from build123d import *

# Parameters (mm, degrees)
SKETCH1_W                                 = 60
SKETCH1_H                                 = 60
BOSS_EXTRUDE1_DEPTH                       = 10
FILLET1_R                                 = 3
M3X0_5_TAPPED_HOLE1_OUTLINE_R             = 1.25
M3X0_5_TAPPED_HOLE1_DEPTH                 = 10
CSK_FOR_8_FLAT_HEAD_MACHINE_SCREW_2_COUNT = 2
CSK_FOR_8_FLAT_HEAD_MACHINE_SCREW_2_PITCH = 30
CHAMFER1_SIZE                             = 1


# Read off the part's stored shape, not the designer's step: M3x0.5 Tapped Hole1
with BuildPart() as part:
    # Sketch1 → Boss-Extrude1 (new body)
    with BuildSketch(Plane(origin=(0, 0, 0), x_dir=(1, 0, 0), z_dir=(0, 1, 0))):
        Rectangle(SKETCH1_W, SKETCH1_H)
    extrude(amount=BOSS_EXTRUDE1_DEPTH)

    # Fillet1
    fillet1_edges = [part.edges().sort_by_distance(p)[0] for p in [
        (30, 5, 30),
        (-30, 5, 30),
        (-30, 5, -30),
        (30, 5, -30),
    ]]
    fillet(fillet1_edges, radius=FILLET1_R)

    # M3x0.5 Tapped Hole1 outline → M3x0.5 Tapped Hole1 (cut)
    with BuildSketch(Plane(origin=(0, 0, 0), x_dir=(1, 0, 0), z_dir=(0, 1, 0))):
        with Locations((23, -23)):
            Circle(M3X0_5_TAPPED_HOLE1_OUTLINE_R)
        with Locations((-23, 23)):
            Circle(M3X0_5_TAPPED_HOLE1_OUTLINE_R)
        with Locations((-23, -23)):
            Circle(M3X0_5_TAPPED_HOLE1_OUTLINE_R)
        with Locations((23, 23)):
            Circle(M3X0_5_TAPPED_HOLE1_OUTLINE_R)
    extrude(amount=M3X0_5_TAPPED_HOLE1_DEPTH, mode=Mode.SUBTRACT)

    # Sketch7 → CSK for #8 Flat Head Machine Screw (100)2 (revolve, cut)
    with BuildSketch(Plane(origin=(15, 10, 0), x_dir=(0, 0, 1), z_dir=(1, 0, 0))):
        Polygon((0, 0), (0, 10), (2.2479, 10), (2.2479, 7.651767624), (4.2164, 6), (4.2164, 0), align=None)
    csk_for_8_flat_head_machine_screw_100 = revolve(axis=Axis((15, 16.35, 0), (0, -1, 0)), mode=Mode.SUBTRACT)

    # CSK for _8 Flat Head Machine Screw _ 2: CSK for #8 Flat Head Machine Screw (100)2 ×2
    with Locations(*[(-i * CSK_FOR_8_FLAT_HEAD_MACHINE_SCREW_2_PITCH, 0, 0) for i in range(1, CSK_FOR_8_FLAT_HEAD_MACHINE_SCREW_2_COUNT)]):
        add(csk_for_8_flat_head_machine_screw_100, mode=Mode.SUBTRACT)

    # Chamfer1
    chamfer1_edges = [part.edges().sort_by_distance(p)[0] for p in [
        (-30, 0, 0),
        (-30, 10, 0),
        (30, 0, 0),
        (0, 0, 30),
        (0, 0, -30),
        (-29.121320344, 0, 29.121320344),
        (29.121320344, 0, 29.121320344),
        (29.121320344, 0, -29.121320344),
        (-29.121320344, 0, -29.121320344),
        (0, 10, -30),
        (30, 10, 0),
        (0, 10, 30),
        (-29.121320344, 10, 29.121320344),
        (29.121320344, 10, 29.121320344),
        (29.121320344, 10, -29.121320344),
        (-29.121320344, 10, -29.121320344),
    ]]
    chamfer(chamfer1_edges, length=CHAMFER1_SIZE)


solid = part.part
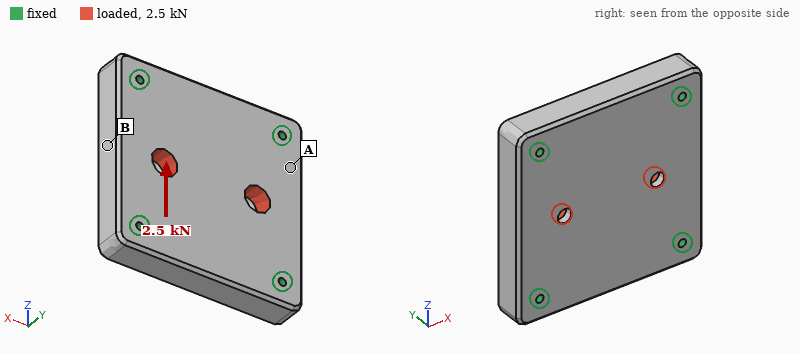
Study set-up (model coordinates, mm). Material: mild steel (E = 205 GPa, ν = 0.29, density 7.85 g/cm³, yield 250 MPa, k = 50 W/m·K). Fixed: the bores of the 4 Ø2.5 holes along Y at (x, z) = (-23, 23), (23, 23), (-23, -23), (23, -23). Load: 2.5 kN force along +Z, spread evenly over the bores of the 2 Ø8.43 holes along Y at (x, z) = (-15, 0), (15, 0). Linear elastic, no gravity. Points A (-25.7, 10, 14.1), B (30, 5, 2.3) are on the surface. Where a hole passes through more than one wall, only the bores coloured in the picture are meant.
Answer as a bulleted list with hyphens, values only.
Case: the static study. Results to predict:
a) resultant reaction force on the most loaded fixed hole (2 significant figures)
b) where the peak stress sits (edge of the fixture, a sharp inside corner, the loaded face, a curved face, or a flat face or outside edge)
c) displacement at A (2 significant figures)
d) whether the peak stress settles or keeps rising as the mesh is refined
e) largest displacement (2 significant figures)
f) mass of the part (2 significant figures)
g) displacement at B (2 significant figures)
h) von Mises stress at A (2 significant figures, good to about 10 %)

- 650 N
- edge of the fixture
- 0.19 µm
- keeps rising
- 0.75 µm
- 270 g
- 0.25 µm
- 3.8 MPa
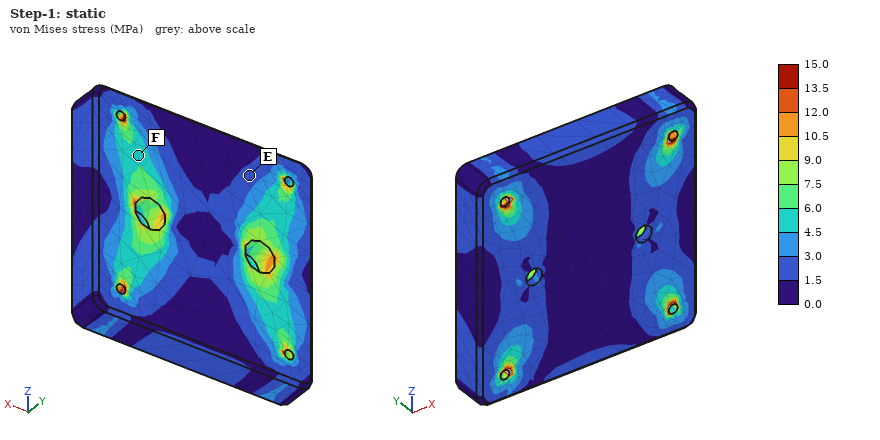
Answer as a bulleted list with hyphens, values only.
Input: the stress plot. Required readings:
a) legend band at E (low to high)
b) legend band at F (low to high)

- 1.5 to 3.0 MPa
- 4.5 to 6.0 MPa
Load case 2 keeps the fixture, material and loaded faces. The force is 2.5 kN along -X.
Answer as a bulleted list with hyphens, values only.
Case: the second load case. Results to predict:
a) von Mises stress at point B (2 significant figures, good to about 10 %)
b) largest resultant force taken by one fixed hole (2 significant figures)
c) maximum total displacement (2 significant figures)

- 5.7 MPa
- 680 N
- 1.1 µm
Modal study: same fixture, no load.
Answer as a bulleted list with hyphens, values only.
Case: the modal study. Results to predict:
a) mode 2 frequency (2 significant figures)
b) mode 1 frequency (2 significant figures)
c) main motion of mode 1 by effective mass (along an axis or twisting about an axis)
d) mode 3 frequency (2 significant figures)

- 19 kHz
- 12 kHz
- along Y
- 19 kHz
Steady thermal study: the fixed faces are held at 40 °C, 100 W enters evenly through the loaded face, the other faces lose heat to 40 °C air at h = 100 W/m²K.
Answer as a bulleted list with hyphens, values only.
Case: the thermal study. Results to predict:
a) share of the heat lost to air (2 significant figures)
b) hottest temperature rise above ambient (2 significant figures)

- 21 %
- 58 K
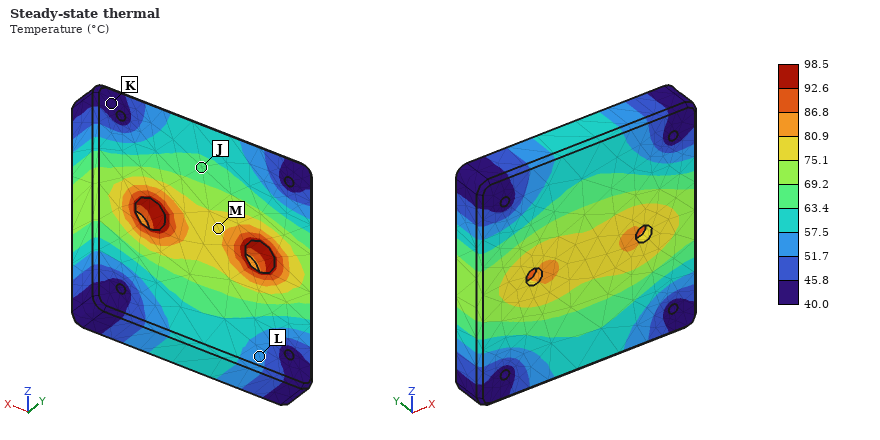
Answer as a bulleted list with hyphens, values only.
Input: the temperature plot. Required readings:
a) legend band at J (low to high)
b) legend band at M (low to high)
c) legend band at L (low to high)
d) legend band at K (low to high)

- 63.4 to 69.2 °C
- 75.1 to 80.9 °C
- 51.7 to 57.5 °C
- 40.0 to 45.8 °C
